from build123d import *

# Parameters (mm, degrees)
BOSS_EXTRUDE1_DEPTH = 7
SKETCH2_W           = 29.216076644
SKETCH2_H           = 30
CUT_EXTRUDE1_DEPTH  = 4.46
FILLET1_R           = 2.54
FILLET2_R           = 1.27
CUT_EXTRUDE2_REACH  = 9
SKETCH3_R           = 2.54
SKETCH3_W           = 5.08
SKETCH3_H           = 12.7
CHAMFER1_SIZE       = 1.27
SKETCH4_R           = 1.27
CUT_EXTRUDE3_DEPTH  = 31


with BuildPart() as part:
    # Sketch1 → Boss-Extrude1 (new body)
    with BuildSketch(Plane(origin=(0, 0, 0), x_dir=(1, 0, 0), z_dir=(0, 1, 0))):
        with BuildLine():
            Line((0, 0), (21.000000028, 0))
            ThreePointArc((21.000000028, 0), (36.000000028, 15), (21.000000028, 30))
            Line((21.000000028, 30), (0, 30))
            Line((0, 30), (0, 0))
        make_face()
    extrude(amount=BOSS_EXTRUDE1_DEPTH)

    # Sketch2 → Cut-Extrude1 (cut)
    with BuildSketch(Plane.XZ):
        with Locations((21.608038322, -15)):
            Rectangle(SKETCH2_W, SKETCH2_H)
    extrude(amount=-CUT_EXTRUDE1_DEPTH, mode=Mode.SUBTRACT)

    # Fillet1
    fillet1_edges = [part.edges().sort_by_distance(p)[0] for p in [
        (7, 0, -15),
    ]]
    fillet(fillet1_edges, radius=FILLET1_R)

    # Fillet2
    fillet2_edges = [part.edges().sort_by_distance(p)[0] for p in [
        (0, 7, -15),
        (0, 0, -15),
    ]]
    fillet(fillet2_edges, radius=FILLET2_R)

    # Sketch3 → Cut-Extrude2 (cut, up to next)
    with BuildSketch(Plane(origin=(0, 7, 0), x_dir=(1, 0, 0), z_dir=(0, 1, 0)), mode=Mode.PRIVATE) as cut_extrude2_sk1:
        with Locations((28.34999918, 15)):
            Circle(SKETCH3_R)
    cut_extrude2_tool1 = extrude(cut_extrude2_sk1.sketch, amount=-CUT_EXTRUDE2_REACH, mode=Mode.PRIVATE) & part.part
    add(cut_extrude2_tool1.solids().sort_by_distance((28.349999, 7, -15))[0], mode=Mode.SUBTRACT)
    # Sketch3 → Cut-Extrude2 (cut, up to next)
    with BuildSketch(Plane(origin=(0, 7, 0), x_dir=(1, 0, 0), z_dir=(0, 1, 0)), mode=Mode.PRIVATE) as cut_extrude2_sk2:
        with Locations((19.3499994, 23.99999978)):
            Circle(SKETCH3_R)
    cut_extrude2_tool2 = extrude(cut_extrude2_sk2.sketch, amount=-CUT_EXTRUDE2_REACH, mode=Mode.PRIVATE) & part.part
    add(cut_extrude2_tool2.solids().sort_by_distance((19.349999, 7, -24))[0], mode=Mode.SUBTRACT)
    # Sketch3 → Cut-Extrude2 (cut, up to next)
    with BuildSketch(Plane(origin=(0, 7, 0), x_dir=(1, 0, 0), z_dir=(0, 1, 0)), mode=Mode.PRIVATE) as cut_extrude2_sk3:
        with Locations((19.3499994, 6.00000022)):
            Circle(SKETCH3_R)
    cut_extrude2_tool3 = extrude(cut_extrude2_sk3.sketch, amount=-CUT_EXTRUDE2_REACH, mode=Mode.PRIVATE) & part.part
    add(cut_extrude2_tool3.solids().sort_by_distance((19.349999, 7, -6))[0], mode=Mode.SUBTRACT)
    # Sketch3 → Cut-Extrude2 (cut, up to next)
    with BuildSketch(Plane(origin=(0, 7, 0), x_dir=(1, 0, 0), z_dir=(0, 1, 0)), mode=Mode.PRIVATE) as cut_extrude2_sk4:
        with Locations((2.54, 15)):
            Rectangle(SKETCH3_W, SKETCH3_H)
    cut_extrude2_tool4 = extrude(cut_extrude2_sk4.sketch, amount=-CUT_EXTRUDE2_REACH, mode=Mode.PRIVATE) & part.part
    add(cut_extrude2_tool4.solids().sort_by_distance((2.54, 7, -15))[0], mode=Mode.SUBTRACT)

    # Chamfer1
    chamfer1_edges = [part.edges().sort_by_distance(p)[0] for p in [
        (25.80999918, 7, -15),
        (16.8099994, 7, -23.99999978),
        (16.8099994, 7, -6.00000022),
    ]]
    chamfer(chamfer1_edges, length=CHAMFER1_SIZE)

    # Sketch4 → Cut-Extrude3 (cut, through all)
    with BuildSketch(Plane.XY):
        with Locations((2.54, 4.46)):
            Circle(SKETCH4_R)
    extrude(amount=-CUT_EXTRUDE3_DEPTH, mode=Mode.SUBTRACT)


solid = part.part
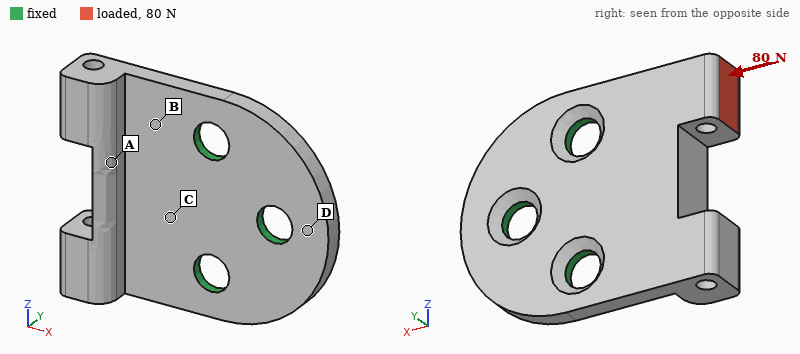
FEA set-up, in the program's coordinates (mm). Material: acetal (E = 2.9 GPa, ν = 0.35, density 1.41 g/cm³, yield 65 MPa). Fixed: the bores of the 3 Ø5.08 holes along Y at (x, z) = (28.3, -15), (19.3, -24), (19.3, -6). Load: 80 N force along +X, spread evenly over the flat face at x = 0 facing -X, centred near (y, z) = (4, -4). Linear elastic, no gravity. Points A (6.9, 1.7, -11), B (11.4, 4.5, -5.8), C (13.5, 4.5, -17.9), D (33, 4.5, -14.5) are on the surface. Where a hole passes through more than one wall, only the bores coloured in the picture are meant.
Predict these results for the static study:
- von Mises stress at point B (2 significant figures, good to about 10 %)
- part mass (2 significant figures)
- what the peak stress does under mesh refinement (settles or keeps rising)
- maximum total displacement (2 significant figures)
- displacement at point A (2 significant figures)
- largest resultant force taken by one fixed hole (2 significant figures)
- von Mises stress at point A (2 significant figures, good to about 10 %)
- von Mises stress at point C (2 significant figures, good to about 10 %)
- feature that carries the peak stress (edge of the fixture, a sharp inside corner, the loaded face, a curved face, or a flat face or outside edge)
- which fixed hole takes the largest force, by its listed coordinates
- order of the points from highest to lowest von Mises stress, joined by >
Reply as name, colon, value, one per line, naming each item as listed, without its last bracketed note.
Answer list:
von Mises stress at point B: 11 MPa
part mass: 3.7 g
what the peak stress does under mesh refinement: keeps rising
maximum total displacement: 0.41 mm
displacement at point A: 0.16 mm
largest resultant force taken by one fixed hole: 81 N
von Mises stress at point A: 6.9 MPa
von Mises stress at point C: 3.7 MPa
feature that carries the peak stress: edge of the fixture
which fixed hole takes the largest force, by its listed coordinates: (19.3, -6)
order of the points from highest to lowest von Mises stress, joined by >: B > A > C > D
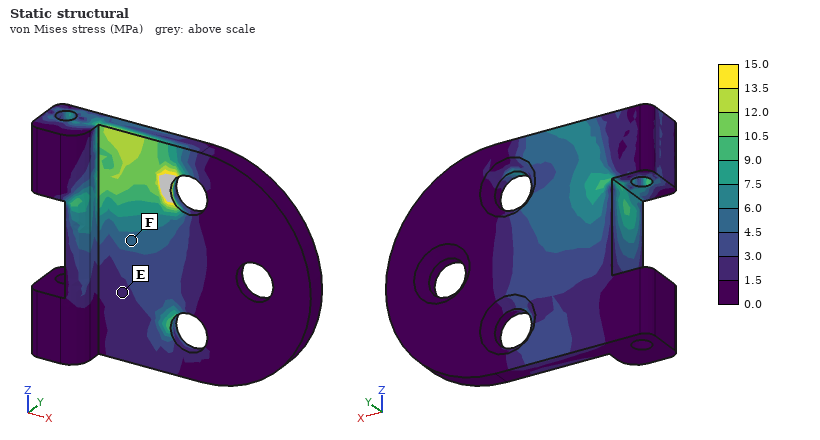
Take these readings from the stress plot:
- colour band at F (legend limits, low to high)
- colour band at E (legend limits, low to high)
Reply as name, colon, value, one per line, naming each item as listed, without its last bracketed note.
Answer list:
colour band at F: 4.5 to 6.0 MPa
colour band at E: 1.5 to 3.0 MPa
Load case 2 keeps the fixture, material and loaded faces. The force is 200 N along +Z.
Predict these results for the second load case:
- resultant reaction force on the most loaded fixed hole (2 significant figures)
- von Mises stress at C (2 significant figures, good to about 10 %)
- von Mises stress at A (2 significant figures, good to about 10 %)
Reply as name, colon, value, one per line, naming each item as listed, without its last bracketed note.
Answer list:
resultant reaction force on the most loaded fixed hole: 210 N
von Mises stress at C: 15 MPa
von Mises stress at A: 7.5 MPa
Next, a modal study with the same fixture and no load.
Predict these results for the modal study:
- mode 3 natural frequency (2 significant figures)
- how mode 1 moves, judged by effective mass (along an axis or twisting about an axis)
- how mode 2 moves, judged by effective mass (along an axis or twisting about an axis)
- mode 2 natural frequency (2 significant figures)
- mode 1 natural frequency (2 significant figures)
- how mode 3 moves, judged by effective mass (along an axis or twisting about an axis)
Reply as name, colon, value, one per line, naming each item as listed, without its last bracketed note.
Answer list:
mode 3 natural frequency: 5800 Hz
how mode 1 moves, judged by effective mass: along Y
how mode 2 moves, judged by effective mass: twisting about X
mode 2 natural frequency: 1800 Hz
mode 1 natural frequency: 1300 Hz
how mode 3 moves, judged by effective mass: along Z
